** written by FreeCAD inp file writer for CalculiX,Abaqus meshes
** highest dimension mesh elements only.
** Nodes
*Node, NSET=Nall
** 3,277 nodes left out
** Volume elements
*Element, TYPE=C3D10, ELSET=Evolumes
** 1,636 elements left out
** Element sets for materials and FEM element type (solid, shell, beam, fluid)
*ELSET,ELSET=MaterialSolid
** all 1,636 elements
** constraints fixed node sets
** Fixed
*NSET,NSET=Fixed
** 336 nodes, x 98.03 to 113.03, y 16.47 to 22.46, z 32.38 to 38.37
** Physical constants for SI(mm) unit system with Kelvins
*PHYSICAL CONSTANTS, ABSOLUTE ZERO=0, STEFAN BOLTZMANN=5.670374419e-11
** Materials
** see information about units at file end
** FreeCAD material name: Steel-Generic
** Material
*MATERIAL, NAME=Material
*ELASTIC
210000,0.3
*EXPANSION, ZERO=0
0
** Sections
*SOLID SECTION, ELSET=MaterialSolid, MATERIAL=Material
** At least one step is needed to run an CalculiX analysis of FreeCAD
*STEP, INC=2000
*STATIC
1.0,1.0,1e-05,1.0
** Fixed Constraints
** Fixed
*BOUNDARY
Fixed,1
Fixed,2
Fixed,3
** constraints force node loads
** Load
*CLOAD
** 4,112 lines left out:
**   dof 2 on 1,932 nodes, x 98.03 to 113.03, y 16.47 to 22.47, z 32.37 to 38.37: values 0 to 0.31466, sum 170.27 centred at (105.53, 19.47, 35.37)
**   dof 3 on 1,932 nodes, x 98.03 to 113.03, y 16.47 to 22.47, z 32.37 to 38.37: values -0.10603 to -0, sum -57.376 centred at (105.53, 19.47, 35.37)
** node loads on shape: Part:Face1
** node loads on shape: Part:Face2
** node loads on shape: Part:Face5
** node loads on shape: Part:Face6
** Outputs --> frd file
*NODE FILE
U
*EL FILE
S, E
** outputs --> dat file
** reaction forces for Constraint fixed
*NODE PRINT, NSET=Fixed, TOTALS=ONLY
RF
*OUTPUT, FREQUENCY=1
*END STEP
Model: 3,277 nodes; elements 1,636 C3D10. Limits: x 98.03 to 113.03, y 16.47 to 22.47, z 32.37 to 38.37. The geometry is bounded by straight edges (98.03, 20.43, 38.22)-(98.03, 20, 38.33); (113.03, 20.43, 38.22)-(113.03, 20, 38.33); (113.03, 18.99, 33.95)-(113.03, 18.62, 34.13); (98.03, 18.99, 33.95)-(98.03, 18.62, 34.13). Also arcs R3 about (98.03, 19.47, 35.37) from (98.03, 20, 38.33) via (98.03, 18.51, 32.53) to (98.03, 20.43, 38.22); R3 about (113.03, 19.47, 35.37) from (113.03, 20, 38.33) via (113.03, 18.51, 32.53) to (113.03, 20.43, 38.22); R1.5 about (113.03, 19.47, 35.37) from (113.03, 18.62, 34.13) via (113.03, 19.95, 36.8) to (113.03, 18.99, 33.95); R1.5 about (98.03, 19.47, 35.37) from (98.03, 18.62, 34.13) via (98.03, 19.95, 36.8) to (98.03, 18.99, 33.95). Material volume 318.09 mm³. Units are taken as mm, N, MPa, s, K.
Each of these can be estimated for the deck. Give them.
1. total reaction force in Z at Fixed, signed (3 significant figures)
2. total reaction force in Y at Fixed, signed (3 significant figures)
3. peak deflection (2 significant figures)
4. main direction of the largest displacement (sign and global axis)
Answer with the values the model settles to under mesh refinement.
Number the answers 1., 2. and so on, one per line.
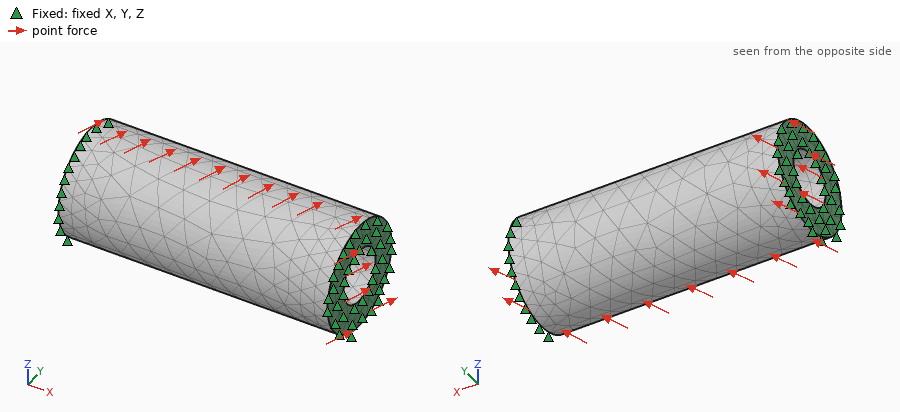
1. 57.4 N
2. -170 N
3. 4.2e-04 mm
4. +Y
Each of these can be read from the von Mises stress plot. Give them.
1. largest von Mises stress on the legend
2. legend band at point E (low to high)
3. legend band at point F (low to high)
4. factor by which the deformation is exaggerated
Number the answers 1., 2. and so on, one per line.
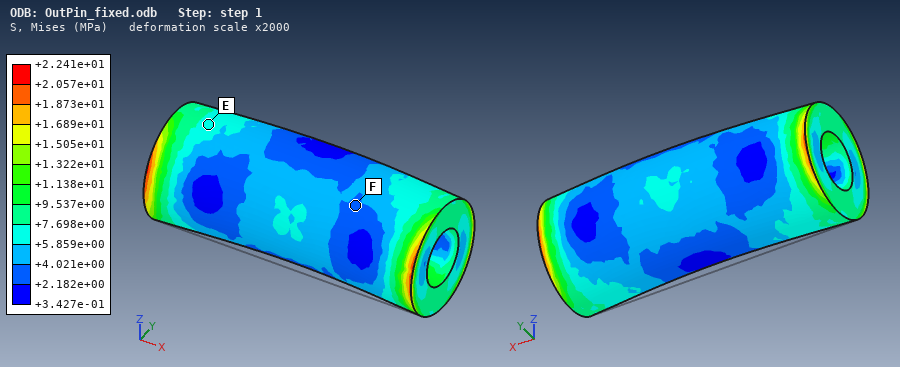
1. +2.241e+01 MPa
2. +5.859e+00 to +7.698e+00 MPa
3. +2.182e+00 to +4.021e+00 MPa
4. 2000
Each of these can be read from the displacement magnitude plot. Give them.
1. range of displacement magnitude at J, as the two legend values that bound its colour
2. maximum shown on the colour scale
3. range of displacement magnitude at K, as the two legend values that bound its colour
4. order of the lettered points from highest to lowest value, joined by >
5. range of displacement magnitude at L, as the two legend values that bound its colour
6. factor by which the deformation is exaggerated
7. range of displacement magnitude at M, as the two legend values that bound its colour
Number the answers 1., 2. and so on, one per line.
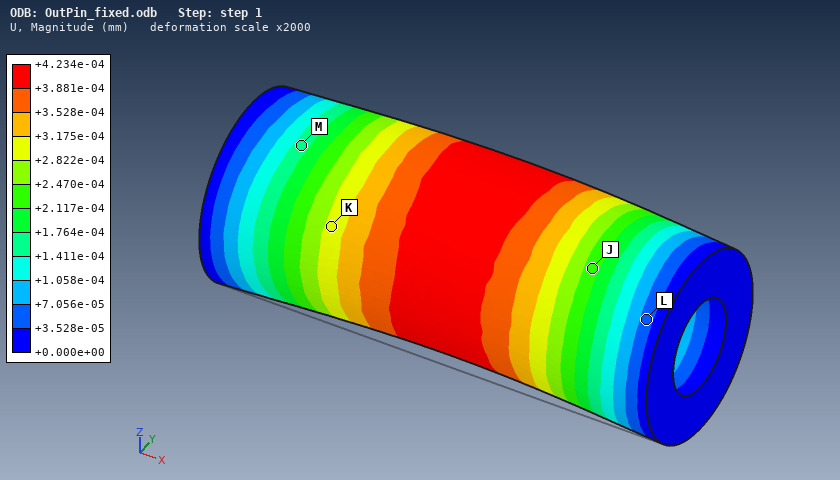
1. +2.117e-04 to +2.470e-04 mm
2. +4.234e-04 mm
3. +2.822e-04 to +3.175e-04 mm
4. K > J > M > L
5. +3.528e-05 to +7.056e-05 mm
6. 2000
7. +1.411e-04 to +1.764e-04 mm
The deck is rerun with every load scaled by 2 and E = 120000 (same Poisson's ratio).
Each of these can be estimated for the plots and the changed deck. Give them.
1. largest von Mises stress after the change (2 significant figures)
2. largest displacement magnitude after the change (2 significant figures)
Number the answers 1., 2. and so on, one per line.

1. 45 MPa
2. 0.0015 mm
